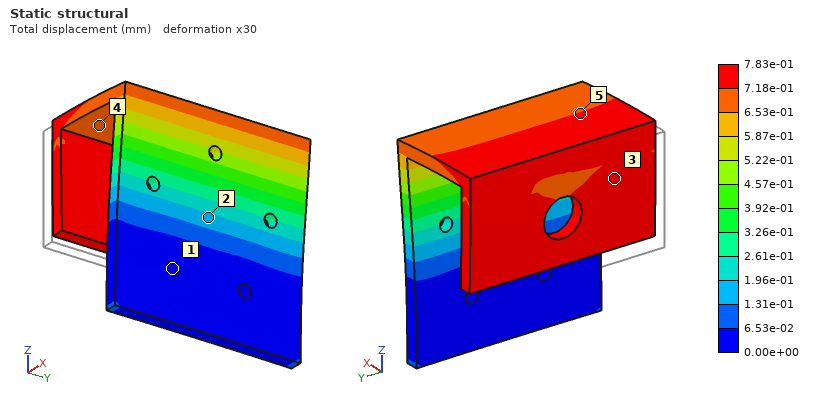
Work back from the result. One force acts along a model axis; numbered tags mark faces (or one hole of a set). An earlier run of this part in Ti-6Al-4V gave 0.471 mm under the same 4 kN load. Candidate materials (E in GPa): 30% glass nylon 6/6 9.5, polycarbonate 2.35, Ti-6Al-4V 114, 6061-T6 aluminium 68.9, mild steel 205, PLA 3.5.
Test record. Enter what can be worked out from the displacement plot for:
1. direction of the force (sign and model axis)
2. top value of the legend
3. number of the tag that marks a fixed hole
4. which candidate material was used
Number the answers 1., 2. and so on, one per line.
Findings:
1. +X
2. 7.83e-01 mm
3. 1
4. 6061-T6 aluminium
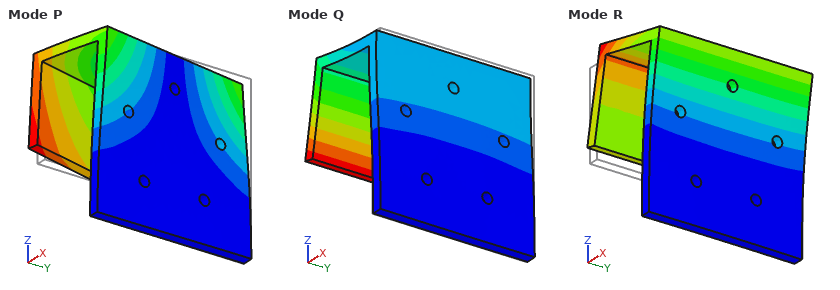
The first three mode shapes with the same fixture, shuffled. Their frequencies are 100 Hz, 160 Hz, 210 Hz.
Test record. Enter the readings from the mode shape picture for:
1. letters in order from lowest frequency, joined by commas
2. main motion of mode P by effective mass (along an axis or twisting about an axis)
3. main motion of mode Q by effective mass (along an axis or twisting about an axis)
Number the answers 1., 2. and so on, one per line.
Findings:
1. R, P, Q
2. along Y
3. along X
